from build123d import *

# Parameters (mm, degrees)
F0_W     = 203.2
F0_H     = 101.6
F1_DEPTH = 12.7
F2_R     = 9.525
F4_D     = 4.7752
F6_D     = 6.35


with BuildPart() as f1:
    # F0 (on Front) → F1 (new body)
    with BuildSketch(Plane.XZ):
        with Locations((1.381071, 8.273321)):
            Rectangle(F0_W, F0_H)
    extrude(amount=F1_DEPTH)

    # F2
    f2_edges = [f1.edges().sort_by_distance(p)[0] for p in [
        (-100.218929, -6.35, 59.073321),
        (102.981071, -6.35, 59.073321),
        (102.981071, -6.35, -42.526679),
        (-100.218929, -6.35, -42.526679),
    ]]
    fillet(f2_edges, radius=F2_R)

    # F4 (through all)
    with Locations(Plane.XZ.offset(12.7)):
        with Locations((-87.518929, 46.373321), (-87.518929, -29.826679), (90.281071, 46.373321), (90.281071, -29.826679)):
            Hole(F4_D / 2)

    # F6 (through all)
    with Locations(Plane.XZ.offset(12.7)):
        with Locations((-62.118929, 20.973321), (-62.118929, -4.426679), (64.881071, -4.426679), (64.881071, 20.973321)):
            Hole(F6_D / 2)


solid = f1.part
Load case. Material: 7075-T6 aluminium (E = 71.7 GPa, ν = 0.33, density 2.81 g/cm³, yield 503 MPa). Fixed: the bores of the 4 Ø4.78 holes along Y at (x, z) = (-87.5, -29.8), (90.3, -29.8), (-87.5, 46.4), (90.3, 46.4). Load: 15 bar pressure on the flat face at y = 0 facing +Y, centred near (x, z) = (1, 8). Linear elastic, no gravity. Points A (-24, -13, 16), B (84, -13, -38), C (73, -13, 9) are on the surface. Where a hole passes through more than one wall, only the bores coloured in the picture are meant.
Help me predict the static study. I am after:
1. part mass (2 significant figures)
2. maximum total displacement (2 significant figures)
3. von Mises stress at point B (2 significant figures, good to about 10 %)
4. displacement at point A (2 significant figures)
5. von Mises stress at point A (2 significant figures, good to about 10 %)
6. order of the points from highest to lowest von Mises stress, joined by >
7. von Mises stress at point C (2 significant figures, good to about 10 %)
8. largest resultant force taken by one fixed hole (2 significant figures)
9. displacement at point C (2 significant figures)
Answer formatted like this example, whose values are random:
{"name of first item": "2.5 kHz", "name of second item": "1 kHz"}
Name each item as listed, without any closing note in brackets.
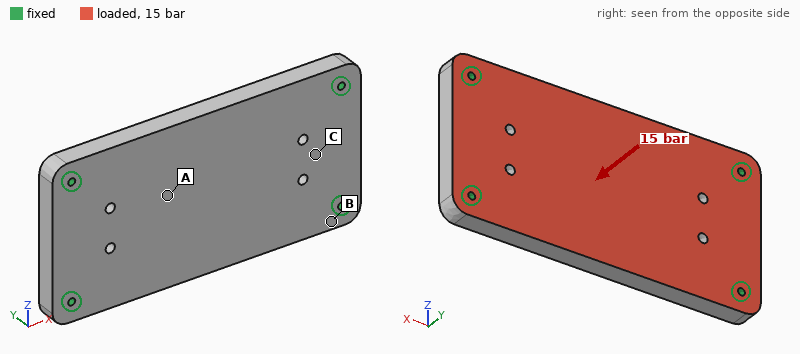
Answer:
{"part mass": "730 g", "maximum total displacement": "0.49 mm", "von Mises stress at point B": "120 MPa", "displacement at point A": "0.41 mm", "von Mises stress at point A": "63 MPa", "order of the points from highest to lowest von Mises stress, joined by >": "B > A > C", "von Mises stress at point C": "38 MPa", "largest resultant force taken by one fixed hole": "7.6 kN", "displacement at point C": "0.13 mm"}
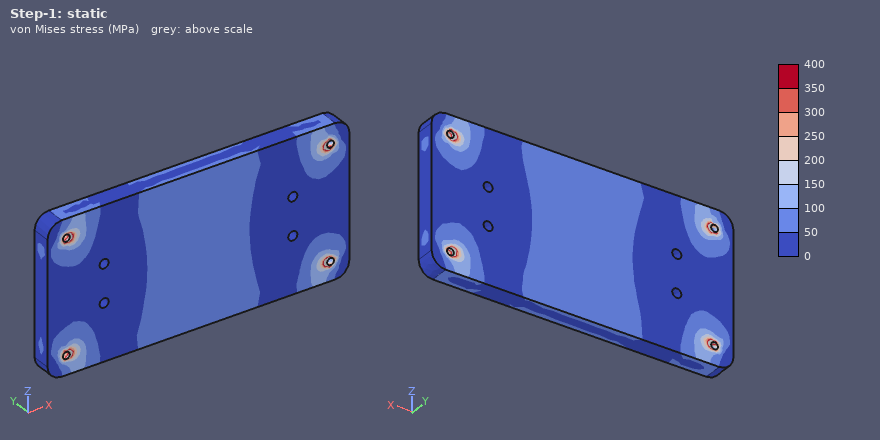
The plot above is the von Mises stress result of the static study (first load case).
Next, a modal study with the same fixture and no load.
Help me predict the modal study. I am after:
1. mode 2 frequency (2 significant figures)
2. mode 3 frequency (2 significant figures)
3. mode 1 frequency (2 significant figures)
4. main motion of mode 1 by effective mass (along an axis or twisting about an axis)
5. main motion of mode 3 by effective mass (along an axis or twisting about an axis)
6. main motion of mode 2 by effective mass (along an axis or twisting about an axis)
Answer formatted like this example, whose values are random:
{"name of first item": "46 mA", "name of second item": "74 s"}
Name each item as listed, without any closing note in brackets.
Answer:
{"mode 2 frequency": "2800 Hz", "mode 3 frequency": "4600 Hz", "mode 1 frequency": "1700 Hz", "main motion of mode 1 by effective mass": "along Y", "main motion of mode 3 by effective mass": "twisting about Z", "main motion of mode 2 by effective mass": "twisting about X"}
